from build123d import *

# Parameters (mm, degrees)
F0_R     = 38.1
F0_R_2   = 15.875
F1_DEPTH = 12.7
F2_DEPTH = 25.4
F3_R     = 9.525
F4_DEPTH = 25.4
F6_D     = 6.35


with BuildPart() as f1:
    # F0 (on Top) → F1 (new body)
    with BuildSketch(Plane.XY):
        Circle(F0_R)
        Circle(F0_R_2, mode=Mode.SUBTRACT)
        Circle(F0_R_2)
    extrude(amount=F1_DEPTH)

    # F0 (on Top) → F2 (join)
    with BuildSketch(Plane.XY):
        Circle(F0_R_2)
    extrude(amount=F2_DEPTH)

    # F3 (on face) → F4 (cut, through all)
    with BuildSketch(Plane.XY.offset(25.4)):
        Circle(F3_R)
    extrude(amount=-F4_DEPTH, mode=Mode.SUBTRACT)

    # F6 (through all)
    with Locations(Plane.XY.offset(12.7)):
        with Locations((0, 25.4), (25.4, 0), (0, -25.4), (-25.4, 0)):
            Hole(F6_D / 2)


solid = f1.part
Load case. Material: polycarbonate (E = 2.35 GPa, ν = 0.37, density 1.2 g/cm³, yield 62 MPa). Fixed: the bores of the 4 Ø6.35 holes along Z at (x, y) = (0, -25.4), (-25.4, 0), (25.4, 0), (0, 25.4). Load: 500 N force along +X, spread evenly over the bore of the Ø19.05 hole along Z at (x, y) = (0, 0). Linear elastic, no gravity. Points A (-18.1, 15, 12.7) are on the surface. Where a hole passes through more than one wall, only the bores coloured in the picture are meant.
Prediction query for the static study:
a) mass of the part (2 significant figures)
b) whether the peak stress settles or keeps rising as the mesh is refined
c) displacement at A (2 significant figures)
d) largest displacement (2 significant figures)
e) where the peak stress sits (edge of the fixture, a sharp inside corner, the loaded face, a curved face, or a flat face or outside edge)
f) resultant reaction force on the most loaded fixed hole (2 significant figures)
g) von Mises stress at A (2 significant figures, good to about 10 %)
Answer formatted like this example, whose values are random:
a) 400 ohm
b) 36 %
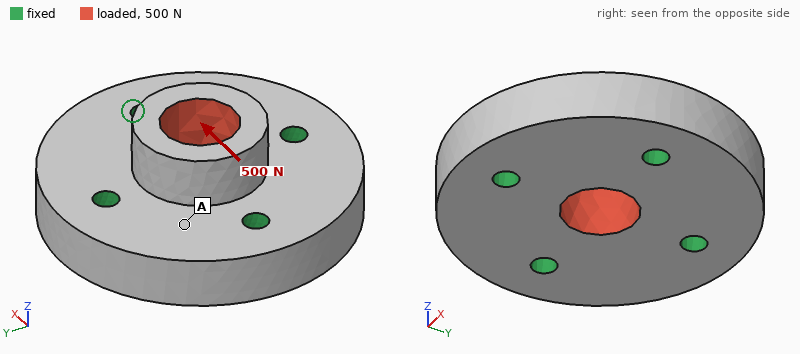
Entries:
a) 71 g
b) keeps rising
c) 3.2 µm
d) 18 µm
e) edge of the fixture
f) 170 N
g) 0.25 MPa
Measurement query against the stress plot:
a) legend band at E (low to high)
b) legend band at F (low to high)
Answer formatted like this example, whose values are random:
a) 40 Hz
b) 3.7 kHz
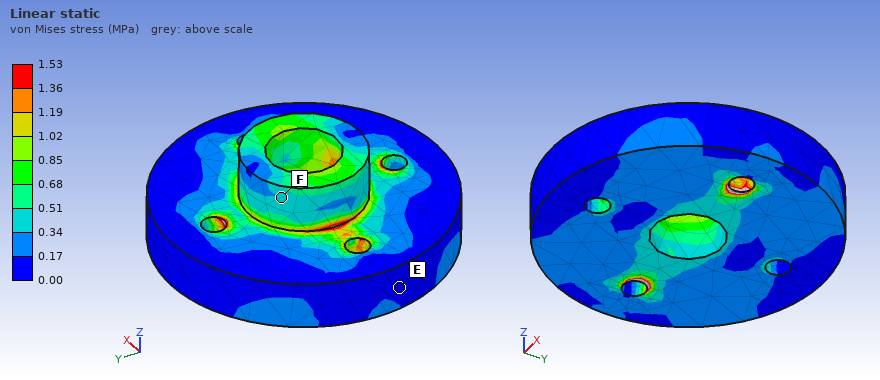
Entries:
a) 0.00 to 0.17 MPa
b) 0.34 to 0.51 MPa
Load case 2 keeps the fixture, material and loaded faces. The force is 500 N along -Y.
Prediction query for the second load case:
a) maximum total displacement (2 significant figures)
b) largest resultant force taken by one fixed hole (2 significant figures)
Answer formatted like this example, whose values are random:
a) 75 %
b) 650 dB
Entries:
a) 18 µm
b) 170 N
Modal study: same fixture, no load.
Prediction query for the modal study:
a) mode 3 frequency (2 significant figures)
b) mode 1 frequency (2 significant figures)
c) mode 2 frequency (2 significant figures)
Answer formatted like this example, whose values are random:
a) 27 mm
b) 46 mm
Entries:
a) 5700 Hz
b) 5400 Hz
c) 5700 Hz
